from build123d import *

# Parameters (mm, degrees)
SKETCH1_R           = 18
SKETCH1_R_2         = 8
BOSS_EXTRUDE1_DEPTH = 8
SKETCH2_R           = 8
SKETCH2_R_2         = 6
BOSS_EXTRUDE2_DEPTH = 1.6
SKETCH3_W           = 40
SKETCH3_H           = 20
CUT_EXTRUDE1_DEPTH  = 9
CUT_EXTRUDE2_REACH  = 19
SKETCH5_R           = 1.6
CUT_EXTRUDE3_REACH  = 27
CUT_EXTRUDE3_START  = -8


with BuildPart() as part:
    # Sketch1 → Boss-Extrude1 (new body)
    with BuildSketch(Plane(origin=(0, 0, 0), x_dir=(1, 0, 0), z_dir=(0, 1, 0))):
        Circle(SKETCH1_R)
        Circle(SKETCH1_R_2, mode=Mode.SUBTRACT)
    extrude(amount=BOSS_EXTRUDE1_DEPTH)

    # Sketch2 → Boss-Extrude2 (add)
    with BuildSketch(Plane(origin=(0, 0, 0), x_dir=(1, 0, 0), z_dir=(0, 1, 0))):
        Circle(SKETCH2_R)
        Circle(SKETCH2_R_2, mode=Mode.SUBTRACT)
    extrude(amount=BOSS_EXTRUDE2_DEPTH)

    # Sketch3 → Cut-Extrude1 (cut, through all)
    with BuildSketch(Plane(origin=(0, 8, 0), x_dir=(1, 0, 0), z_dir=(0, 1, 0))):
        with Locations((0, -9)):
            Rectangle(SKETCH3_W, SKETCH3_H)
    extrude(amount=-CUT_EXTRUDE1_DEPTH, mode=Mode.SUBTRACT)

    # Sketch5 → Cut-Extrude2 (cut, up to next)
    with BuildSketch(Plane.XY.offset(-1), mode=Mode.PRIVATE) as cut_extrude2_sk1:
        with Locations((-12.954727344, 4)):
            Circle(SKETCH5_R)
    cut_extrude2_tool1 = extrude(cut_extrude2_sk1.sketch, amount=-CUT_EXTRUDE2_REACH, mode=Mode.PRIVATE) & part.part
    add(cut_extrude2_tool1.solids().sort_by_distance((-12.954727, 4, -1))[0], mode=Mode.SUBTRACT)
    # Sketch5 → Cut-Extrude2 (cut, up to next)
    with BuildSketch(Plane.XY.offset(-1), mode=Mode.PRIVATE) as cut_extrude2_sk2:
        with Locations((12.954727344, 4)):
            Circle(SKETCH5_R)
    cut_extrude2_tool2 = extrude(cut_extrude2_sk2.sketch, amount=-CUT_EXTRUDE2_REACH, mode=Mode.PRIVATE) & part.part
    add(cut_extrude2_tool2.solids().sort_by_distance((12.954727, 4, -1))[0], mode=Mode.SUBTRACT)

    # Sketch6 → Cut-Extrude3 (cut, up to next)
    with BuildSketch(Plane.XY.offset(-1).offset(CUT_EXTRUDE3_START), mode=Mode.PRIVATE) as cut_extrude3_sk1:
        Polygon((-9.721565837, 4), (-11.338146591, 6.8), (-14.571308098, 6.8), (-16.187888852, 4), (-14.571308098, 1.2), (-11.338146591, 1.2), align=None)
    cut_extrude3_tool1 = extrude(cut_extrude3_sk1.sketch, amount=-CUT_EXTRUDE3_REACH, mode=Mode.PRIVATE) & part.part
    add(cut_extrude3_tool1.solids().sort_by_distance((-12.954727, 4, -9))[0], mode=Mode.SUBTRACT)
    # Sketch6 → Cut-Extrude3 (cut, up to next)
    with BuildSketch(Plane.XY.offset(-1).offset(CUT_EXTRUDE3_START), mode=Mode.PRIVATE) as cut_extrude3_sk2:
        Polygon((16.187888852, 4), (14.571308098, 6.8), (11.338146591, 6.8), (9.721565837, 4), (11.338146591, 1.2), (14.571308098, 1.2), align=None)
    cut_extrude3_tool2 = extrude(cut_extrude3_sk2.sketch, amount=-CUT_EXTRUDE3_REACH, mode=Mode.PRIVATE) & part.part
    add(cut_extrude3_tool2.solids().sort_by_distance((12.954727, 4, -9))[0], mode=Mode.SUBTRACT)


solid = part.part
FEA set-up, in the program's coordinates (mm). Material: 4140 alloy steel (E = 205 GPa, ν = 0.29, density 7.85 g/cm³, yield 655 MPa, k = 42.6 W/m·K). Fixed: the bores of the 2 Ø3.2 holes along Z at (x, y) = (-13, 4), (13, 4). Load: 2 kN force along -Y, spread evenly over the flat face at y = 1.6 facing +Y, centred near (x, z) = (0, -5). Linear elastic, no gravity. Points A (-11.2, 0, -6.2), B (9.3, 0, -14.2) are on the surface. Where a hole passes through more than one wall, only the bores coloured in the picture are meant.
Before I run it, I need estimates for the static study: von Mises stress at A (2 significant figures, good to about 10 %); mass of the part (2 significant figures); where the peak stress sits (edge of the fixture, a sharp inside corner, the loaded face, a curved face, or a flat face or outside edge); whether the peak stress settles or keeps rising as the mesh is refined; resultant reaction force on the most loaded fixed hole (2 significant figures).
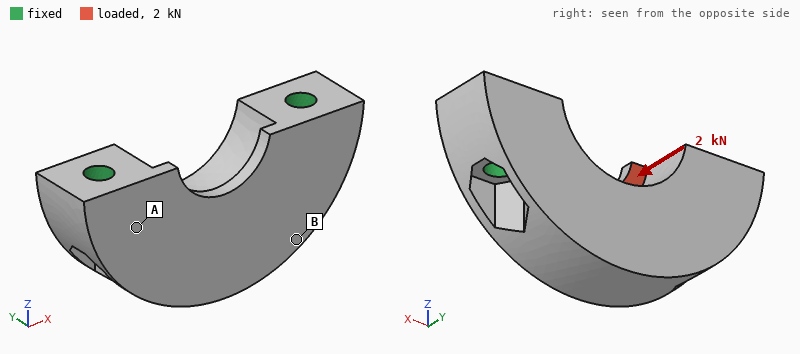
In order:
37 MPa
22 g
a sharp inside corner
keeps rising
1.0 kN
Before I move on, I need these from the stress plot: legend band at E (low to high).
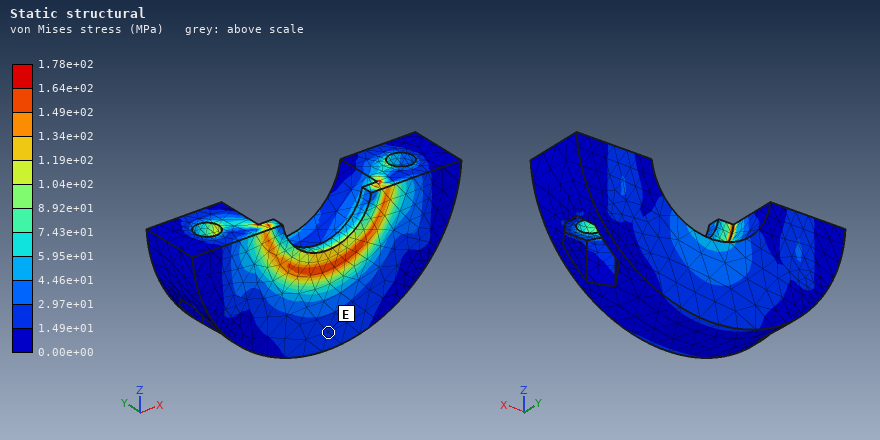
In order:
1.49e+01 to 2.97e+01 MPa
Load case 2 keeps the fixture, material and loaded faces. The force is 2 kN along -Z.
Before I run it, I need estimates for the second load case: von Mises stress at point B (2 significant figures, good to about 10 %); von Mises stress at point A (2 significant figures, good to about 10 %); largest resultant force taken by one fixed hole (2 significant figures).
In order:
22 MPa
41 MPa
1.1 kN
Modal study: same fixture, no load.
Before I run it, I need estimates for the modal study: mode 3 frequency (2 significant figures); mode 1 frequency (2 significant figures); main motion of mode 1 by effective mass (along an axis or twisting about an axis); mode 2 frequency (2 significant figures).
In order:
51 kHz
22 kHz
along Y
49 kHz
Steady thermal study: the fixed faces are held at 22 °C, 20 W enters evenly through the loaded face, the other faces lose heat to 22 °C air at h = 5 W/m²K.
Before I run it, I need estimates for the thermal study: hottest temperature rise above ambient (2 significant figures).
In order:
59 K
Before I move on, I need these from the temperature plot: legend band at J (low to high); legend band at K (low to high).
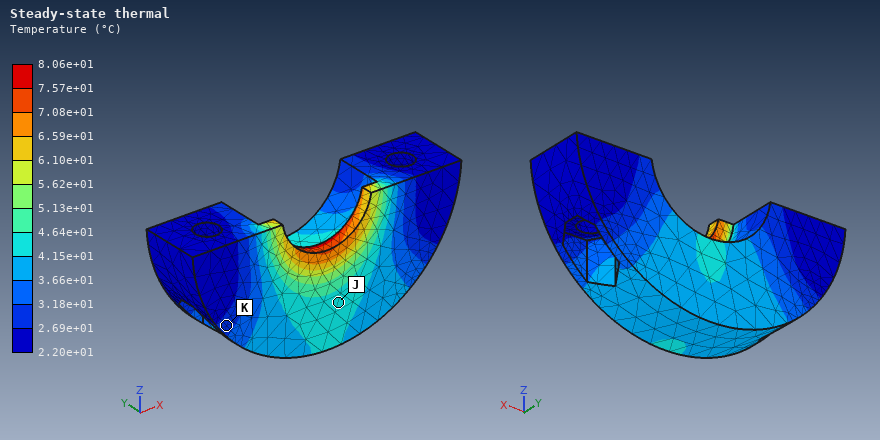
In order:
4.15e+01 to 4.64e+01 °C
2.69e+01 to 3.18e+01 °C
